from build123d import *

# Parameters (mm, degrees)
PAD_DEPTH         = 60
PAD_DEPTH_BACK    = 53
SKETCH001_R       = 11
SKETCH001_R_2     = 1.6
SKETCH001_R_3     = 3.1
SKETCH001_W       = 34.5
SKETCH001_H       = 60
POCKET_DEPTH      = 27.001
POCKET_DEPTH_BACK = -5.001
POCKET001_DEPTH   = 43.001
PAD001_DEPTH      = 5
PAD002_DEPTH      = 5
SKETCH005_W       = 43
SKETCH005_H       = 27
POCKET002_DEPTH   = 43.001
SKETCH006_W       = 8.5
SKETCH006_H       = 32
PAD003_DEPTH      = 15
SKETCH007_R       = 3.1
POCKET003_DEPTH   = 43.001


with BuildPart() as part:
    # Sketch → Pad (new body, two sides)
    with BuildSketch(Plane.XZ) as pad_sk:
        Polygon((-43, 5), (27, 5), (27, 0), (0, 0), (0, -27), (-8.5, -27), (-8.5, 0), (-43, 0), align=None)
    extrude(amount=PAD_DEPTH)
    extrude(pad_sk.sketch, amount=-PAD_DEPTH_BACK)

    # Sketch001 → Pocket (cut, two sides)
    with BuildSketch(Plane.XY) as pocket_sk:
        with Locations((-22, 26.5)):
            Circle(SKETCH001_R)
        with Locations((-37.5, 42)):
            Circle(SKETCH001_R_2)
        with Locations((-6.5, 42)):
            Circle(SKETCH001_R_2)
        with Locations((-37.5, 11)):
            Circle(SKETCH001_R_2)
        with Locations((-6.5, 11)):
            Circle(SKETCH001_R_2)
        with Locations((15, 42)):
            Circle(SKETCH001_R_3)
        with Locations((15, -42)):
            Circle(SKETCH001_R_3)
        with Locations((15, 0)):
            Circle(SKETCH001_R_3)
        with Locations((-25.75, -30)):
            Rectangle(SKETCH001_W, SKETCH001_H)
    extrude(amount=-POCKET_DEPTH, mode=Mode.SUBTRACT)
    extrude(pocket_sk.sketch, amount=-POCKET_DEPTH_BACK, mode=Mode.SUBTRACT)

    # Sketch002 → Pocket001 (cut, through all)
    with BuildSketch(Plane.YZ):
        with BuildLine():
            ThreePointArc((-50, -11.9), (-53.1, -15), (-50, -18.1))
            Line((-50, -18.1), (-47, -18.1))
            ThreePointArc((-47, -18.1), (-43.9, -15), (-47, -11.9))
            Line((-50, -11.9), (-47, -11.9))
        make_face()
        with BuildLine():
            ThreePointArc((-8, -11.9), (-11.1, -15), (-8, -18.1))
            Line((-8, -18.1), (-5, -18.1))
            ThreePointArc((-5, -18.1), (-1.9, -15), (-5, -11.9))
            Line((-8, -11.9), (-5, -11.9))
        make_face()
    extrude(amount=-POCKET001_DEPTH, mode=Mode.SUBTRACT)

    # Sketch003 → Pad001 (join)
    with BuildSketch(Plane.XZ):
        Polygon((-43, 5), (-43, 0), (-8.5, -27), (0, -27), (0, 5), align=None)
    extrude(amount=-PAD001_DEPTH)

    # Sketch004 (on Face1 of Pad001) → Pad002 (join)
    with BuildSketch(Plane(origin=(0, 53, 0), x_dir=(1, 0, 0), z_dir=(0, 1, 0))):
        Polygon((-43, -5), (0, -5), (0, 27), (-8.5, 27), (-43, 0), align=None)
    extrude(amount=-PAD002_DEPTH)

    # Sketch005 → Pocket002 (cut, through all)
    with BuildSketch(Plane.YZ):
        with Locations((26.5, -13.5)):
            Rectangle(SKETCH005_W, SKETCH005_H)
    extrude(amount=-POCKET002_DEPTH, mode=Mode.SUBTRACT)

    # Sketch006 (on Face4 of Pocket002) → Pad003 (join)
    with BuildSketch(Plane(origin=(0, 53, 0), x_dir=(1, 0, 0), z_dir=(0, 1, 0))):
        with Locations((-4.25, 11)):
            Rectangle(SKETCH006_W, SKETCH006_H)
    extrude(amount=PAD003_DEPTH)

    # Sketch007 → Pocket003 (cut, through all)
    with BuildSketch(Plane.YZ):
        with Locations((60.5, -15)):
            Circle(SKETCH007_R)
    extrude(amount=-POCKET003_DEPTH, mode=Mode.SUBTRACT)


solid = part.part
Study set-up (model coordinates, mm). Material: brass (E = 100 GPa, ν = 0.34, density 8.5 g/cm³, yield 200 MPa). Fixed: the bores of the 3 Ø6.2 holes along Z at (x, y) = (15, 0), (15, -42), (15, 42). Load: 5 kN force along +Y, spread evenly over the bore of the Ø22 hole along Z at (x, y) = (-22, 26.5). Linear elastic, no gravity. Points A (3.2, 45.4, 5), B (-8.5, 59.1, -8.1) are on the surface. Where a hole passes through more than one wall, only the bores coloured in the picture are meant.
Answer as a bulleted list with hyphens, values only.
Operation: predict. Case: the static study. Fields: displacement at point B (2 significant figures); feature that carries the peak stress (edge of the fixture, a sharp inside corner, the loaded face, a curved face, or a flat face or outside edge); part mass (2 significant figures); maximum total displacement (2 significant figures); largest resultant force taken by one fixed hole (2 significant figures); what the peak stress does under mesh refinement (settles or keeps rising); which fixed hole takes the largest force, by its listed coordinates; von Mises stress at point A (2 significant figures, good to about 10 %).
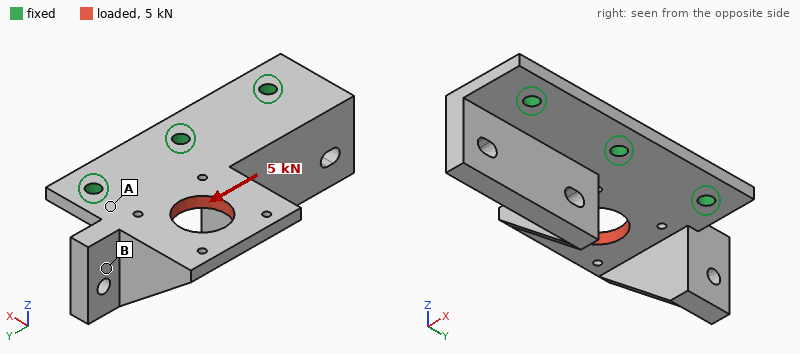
- 31 µm
- edge of the fixture
- 430 g
- 56 µm
- 3.6 kN
- keeps rising
- (15, 42)
- 21 MPa
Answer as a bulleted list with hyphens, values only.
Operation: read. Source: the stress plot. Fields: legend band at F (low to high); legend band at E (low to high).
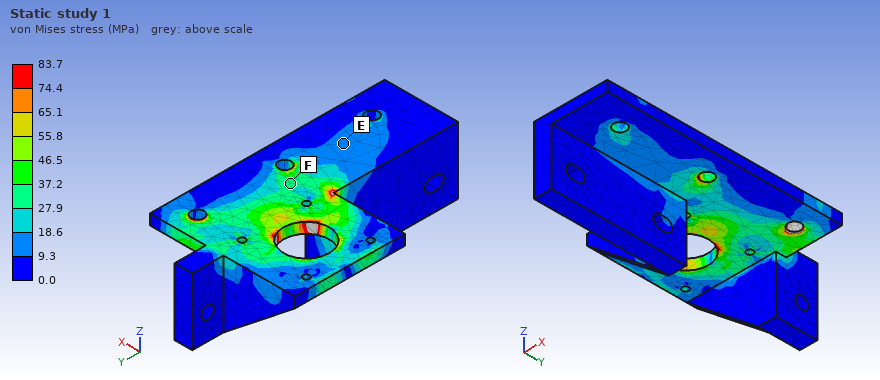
- 27.9 to 37.2 MPa
- 9.3 to 18.6 MPa
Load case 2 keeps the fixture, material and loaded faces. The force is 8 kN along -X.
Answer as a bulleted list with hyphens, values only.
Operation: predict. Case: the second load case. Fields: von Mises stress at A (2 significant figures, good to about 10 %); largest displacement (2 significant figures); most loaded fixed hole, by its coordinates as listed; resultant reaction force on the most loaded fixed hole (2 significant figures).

- 42 MPa
- 30 µm
- (15, 42)
- 5.1 kN
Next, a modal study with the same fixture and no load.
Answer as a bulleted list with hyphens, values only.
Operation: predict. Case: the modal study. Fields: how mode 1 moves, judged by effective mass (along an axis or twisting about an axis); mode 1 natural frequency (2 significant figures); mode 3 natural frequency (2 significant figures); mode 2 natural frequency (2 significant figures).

- along Z
- 840 Hz
- 1900 Hz
- 1200 Hz
